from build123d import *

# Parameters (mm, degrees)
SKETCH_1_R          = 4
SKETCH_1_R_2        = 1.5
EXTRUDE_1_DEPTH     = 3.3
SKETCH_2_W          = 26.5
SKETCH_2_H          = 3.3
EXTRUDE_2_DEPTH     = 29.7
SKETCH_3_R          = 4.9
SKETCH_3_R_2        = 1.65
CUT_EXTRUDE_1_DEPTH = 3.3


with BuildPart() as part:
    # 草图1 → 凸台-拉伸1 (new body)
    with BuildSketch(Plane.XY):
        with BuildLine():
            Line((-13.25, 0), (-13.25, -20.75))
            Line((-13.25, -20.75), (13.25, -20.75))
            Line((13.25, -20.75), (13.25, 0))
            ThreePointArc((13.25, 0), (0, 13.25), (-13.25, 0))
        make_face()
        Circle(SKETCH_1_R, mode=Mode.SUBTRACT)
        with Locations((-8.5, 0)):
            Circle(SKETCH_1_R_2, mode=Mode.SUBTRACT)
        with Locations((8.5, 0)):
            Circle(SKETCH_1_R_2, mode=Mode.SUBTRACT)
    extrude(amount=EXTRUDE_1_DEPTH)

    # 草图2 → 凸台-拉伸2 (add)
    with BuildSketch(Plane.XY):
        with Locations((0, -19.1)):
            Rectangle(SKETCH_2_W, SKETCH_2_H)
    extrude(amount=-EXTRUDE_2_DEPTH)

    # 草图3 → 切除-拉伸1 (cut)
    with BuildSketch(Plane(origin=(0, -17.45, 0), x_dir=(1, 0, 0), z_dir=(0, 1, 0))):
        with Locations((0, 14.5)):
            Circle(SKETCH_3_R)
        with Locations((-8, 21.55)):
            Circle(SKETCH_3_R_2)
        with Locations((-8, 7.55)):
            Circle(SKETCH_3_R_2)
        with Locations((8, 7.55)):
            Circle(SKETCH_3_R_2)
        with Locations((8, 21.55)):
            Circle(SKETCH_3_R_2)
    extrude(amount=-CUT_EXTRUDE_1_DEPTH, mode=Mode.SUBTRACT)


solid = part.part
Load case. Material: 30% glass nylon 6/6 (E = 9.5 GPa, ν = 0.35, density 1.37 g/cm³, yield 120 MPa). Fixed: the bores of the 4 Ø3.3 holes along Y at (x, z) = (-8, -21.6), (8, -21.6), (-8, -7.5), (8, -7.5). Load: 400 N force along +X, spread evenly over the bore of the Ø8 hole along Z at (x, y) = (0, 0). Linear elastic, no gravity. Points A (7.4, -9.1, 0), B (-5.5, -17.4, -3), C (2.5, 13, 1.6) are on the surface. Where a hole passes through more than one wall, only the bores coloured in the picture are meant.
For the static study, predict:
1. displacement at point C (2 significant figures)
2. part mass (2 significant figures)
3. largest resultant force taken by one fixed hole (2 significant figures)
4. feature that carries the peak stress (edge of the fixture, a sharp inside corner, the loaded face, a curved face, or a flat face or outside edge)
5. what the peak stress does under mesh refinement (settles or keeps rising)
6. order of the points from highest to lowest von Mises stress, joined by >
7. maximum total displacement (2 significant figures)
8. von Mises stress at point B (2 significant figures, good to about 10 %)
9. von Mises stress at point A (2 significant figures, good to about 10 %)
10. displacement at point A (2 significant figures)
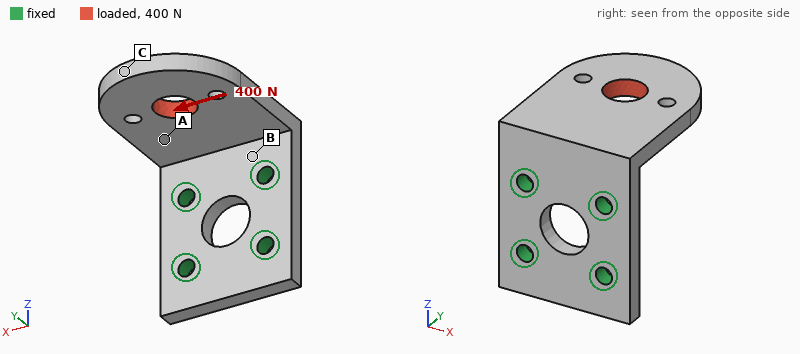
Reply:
0.62 mm
6.5 g
500 N
edge of the fixture
keeps rising
B > A > C
0.65 mm
53 MPa
21 MPa
0.26 mm
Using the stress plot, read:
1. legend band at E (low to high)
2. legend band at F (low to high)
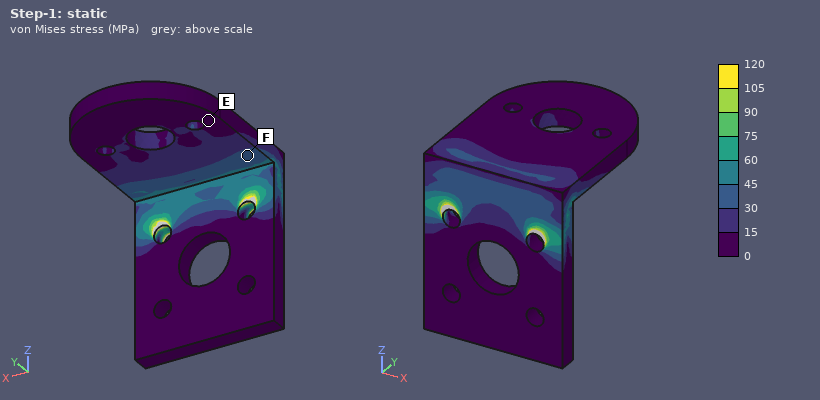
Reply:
0 to 15 MPa
30 to 45 MPa
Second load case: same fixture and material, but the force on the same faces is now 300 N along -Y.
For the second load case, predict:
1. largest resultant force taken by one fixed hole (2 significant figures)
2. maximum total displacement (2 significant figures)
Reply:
160 N
0.52 mm
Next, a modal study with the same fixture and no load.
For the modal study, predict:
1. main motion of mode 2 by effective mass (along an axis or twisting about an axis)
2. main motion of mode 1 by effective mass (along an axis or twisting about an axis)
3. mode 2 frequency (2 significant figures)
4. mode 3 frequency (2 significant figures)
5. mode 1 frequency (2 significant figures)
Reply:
along X
along Z
2800 Hz
4400 Hz
1200 Hz
